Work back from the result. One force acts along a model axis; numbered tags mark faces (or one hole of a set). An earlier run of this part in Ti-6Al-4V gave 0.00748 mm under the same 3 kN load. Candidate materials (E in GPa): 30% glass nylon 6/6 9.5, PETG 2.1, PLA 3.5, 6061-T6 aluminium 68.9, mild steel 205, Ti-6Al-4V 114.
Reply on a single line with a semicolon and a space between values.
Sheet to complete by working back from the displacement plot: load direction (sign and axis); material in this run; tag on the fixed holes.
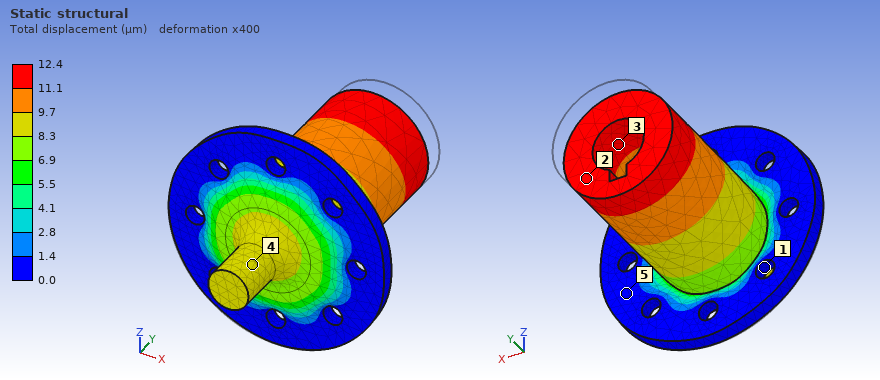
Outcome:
-Y; 6061-T6 aluminium; 1
